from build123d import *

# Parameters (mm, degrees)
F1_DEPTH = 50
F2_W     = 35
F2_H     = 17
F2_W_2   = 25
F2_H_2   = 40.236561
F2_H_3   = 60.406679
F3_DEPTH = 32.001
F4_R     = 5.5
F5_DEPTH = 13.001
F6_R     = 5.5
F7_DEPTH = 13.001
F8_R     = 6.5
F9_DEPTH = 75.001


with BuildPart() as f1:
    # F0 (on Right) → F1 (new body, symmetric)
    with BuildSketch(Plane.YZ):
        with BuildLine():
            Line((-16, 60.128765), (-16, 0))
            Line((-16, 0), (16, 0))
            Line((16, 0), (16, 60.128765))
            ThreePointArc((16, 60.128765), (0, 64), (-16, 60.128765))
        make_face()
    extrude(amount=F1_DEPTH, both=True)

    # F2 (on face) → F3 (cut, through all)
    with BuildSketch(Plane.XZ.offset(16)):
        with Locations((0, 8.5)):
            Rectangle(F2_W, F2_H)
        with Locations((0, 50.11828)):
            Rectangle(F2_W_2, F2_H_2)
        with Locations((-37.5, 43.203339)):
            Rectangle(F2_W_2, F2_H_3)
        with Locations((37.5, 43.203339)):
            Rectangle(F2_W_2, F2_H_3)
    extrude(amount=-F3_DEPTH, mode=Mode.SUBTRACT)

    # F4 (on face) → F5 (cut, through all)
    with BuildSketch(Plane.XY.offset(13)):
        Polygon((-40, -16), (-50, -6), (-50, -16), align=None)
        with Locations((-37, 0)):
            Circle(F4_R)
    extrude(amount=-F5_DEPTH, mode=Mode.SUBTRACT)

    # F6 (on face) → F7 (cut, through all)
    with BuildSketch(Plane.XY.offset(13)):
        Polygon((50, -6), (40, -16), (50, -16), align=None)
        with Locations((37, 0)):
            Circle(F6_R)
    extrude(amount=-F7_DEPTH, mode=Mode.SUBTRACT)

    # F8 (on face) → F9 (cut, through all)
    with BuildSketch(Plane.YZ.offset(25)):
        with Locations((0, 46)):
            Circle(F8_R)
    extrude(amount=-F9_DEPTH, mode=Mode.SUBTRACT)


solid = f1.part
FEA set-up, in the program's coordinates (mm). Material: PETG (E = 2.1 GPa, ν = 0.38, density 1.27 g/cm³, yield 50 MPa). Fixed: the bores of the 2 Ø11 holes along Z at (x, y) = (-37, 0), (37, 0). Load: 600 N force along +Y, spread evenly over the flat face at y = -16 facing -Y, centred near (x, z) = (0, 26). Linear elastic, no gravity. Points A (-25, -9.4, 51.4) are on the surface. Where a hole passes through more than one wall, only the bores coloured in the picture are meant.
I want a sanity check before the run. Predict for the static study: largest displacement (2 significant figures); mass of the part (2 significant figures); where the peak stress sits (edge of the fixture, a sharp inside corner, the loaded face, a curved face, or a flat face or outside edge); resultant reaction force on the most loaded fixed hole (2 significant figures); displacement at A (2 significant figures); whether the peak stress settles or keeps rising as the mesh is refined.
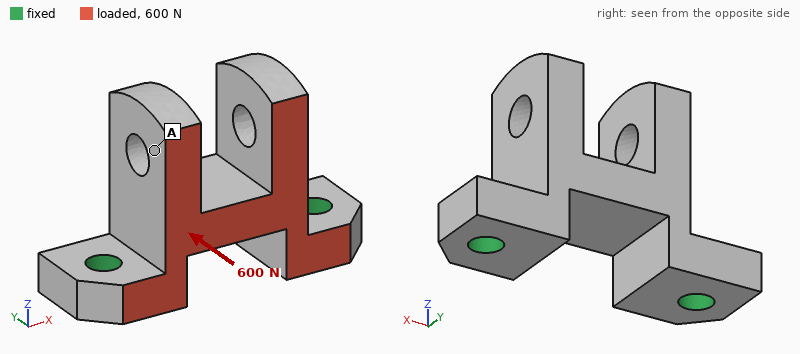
0.39 mm
87 g
edge of the fixture
300 N
0.32 mm
keeps rising
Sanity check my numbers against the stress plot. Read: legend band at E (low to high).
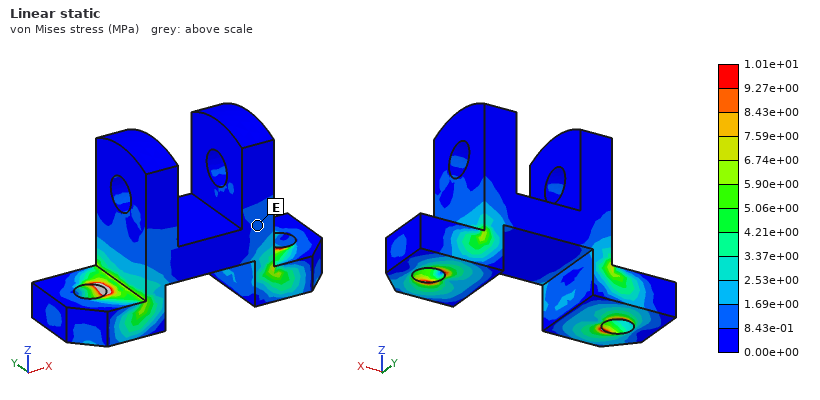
8.43e-01 to 1.69e+00 MPa
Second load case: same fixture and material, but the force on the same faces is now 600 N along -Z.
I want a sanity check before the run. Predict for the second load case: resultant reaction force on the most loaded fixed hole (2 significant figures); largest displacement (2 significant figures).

320 N
0.27 mm
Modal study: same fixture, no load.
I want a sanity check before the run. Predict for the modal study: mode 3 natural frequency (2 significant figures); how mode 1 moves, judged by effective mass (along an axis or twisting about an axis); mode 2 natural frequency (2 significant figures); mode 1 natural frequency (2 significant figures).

1300 Hz
along Y
1300 Hz
840 Hz
